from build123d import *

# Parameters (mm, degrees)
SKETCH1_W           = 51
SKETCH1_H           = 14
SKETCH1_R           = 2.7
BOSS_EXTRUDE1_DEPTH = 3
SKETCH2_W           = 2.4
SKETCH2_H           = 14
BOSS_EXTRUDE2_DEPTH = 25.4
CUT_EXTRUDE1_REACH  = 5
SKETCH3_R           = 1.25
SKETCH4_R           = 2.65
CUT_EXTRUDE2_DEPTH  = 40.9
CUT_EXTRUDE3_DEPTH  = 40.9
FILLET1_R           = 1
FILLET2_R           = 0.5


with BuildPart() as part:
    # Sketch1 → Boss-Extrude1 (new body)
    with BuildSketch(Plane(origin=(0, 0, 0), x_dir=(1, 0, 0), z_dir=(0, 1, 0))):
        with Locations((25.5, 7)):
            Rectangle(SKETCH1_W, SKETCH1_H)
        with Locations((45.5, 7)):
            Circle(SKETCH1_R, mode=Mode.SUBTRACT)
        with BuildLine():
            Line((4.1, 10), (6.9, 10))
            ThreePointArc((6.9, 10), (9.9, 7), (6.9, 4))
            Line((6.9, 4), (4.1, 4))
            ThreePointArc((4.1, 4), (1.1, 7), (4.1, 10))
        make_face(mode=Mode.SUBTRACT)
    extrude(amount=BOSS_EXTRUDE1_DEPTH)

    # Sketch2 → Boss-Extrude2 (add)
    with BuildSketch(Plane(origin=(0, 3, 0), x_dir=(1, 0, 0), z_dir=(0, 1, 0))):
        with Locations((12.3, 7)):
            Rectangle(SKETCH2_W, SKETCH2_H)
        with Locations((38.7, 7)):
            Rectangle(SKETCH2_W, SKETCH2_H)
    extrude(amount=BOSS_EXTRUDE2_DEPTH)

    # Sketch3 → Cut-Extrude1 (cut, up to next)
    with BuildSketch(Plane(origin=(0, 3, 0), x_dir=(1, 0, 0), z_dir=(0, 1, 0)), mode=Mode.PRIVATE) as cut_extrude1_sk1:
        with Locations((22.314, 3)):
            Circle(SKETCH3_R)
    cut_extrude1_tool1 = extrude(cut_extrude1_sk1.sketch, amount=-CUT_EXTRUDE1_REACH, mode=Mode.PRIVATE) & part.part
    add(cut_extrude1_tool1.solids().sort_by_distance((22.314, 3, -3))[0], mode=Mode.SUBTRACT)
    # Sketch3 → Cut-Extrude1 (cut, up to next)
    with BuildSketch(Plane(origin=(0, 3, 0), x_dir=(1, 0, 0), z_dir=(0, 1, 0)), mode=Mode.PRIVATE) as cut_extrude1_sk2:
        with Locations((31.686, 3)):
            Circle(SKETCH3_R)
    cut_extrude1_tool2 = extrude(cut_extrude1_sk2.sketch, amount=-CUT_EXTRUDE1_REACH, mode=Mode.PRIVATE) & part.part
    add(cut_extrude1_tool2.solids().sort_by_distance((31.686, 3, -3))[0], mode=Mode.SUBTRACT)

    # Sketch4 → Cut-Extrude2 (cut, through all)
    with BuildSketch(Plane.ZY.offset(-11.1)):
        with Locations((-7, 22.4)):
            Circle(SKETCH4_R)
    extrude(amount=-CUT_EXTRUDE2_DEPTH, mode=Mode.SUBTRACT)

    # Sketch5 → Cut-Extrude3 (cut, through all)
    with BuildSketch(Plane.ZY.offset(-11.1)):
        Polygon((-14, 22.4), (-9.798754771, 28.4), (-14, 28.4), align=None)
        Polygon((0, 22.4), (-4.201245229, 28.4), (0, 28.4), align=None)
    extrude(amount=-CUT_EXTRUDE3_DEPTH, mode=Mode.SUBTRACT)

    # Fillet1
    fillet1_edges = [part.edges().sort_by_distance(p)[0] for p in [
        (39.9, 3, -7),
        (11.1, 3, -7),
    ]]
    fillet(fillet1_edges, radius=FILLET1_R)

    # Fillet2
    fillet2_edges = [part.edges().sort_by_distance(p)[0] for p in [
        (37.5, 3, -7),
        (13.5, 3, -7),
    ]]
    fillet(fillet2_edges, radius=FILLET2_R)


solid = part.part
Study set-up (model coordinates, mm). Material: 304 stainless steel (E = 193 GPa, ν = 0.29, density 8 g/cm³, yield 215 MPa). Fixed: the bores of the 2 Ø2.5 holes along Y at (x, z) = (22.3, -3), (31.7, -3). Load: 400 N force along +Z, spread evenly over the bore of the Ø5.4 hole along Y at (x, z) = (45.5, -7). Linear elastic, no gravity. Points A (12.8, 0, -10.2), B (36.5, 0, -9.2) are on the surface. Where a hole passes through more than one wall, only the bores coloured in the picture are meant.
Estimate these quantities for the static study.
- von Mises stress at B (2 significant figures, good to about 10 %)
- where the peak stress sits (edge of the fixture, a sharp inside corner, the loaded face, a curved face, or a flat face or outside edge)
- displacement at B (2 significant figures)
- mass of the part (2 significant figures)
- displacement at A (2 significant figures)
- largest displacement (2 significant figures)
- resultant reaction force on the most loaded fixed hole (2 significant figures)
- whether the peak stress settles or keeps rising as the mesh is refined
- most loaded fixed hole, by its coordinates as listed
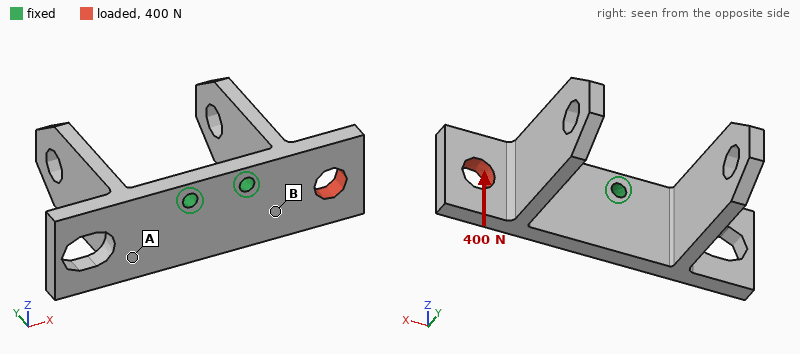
24 MPa
edge of the fixture
3.5 µm
27 g
2.4 µm
14 µm
840 N
keeps rising
(31.7, -3)
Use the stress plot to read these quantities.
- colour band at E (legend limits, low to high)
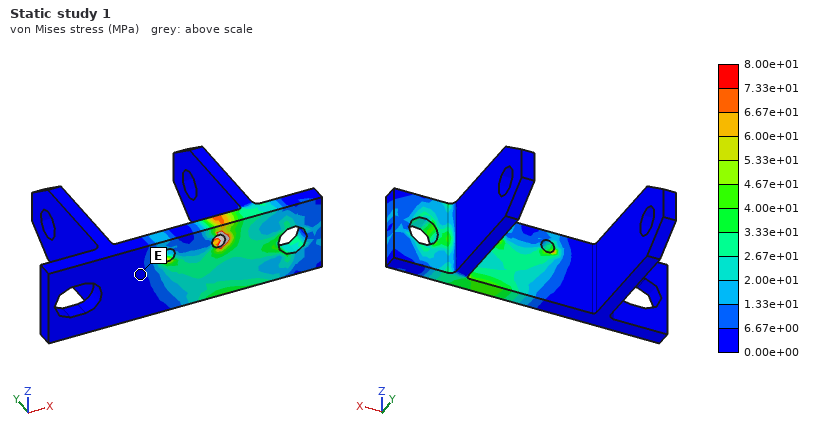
0.00e+00 to 6.67e+00 MPa
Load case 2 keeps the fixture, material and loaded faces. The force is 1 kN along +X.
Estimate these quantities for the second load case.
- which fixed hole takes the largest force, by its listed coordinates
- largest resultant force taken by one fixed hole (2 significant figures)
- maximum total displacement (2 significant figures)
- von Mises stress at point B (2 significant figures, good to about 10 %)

(31.7, -3)
790 N
6.0 µm
23 MPa
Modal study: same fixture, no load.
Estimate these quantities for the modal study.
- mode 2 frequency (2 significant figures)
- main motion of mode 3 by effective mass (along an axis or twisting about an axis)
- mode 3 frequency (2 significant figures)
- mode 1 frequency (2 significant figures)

2600 Hz
along Z
3700 Hz
2300 Hz
